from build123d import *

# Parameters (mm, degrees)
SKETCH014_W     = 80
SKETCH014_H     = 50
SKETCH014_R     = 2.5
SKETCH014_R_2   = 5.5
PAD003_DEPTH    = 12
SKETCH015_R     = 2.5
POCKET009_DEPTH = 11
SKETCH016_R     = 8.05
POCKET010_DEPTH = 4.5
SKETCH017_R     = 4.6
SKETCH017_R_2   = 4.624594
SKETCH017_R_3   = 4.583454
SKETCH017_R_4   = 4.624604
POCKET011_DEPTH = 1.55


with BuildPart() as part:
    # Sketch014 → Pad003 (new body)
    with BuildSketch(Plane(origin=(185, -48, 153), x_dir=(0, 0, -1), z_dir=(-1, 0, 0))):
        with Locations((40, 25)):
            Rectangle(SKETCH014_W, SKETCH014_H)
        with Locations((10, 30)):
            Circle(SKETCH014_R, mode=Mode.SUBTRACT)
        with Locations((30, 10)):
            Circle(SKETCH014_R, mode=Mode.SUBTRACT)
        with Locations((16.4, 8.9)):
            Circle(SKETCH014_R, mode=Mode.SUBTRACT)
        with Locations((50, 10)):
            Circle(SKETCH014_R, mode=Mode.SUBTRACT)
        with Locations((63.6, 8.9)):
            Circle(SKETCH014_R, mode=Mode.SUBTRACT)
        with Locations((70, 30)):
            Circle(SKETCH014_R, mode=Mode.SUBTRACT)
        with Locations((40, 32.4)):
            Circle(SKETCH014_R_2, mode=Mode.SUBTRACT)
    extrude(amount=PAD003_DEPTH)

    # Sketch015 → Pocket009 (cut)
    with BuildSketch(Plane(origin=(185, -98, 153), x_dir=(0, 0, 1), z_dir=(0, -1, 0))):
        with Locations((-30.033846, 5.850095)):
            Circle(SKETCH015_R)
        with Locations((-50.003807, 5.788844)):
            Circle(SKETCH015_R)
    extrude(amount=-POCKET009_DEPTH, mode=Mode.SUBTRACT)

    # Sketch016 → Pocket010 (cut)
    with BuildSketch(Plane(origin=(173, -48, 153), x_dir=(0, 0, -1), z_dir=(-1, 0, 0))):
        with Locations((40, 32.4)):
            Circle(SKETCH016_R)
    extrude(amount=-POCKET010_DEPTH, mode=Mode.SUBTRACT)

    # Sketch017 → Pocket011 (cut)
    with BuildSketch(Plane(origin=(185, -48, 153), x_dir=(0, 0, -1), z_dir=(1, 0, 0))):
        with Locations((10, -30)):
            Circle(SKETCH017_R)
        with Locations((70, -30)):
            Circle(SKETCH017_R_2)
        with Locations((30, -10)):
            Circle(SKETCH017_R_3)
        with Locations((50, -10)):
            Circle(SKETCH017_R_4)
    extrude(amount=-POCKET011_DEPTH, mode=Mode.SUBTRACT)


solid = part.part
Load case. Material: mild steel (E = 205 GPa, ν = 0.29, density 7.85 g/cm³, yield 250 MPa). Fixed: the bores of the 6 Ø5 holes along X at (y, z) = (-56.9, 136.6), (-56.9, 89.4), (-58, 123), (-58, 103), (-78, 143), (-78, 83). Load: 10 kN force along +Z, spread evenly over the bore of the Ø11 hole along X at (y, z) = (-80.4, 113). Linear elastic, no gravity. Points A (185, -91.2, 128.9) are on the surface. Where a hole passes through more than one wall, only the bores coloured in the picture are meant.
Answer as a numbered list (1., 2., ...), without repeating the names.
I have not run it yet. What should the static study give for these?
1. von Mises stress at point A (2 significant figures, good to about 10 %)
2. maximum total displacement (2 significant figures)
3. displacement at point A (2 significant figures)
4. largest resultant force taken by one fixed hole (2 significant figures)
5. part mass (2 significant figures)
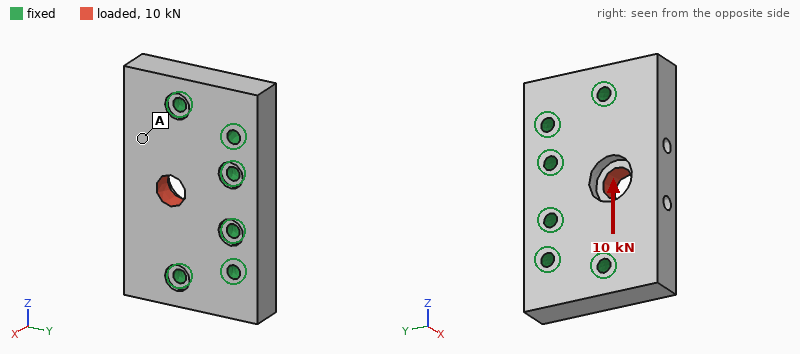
1. 13 MPa
2. 3.9 µm
3. 2.1 µm
4. 3.5 kN
5. 350 g
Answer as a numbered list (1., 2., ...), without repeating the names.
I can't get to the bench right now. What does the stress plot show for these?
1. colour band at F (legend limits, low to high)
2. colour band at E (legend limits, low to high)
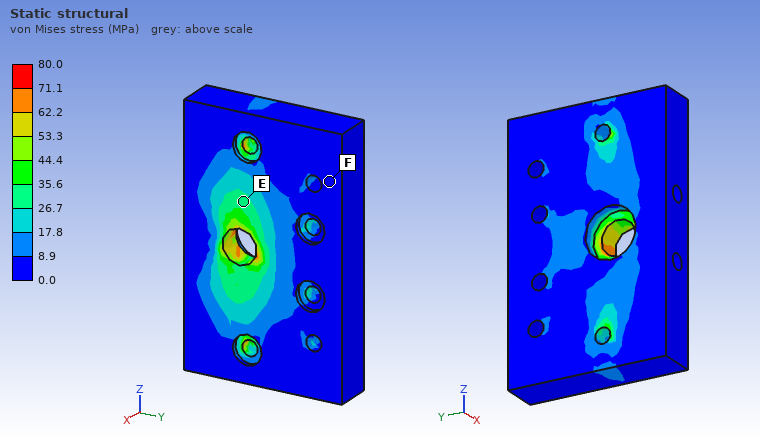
1. 0.0 to 8.9 MPa
2. 26.7 to 35.6 MPa
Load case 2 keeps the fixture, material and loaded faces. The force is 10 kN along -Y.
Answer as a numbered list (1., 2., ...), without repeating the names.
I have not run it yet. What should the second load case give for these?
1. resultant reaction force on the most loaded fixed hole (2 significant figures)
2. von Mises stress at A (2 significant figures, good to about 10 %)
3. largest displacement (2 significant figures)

1. 3.2 kN
2. 14 MPa
3. 6.1 µm
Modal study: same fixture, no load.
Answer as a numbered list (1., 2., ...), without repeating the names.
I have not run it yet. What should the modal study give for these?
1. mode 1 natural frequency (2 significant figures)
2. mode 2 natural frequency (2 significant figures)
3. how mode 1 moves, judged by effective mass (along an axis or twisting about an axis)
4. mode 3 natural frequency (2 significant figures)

1. 12 kHz
2. 18 kHz
3. along X
4. 22 kHz
